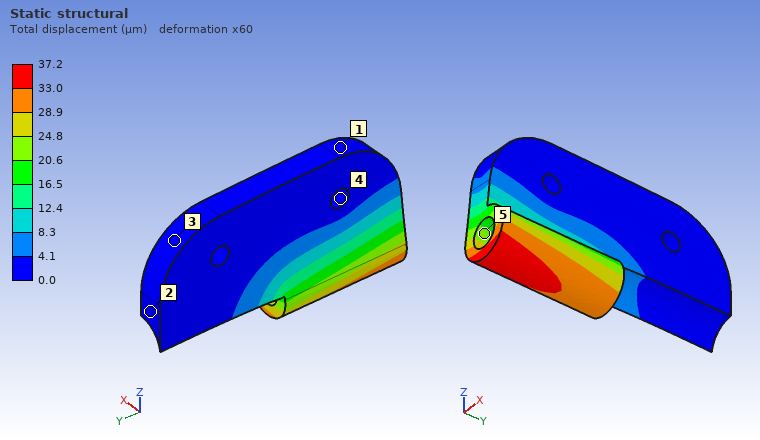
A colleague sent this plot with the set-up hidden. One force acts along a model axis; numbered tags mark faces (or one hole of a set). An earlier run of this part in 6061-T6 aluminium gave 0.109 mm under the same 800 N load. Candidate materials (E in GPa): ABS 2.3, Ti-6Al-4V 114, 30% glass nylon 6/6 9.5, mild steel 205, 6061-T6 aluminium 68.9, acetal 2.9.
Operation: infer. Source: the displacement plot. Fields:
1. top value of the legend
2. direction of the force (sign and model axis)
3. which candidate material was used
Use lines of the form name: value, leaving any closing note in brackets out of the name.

top value of the legend: 37.2 µm
direction of the force: -X
which candidate material was used: mild steel
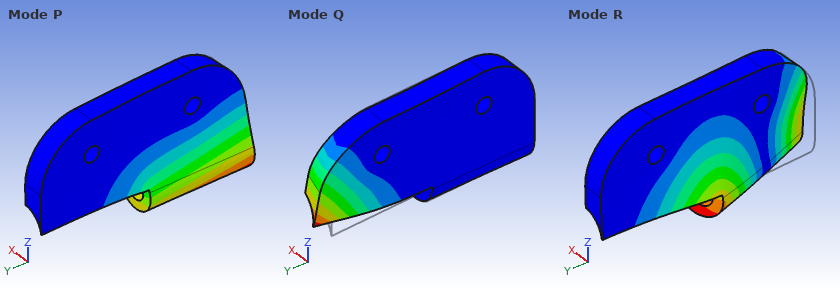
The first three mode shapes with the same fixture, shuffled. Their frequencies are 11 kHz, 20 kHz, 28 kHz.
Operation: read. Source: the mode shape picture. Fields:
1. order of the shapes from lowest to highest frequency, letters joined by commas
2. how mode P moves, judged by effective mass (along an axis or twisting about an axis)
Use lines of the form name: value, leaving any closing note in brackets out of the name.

order of the shapes from lowest to highest frequency, letters joined by commas: P, R, Q
how mode P moves, judged by effective mass: along X
